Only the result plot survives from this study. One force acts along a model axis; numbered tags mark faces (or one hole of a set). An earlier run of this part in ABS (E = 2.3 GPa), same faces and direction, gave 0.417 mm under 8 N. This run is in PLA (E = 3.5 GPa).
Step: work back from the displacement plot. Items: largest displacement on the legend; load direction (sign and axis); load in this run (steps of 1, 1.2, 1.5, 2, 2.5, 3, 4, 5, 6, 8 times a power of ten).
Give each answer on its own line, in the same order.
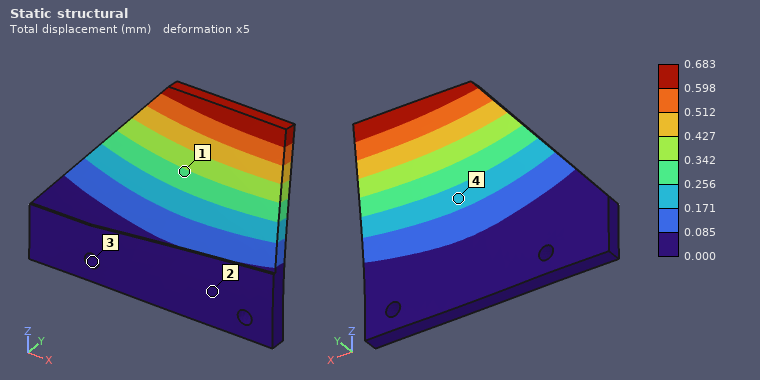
0.683 mm
+Y
20 N
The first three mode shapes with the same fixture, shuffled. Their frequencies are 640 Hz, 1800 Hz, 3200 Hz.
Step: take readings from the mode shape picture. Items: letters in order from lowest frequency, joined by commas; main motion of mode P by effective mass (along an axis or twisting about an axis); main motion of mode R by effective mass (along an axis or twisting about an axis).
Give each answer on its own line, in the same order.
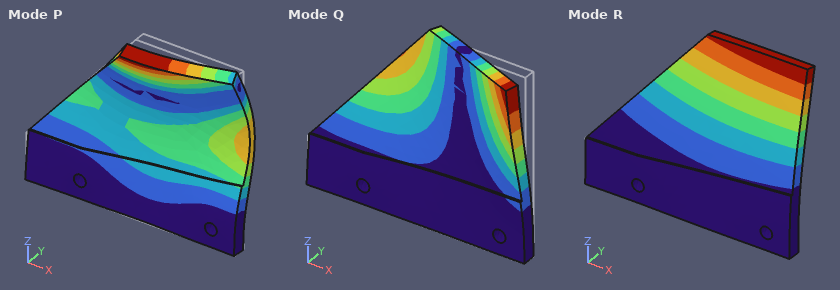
R, Q, P
along Y
along Y
